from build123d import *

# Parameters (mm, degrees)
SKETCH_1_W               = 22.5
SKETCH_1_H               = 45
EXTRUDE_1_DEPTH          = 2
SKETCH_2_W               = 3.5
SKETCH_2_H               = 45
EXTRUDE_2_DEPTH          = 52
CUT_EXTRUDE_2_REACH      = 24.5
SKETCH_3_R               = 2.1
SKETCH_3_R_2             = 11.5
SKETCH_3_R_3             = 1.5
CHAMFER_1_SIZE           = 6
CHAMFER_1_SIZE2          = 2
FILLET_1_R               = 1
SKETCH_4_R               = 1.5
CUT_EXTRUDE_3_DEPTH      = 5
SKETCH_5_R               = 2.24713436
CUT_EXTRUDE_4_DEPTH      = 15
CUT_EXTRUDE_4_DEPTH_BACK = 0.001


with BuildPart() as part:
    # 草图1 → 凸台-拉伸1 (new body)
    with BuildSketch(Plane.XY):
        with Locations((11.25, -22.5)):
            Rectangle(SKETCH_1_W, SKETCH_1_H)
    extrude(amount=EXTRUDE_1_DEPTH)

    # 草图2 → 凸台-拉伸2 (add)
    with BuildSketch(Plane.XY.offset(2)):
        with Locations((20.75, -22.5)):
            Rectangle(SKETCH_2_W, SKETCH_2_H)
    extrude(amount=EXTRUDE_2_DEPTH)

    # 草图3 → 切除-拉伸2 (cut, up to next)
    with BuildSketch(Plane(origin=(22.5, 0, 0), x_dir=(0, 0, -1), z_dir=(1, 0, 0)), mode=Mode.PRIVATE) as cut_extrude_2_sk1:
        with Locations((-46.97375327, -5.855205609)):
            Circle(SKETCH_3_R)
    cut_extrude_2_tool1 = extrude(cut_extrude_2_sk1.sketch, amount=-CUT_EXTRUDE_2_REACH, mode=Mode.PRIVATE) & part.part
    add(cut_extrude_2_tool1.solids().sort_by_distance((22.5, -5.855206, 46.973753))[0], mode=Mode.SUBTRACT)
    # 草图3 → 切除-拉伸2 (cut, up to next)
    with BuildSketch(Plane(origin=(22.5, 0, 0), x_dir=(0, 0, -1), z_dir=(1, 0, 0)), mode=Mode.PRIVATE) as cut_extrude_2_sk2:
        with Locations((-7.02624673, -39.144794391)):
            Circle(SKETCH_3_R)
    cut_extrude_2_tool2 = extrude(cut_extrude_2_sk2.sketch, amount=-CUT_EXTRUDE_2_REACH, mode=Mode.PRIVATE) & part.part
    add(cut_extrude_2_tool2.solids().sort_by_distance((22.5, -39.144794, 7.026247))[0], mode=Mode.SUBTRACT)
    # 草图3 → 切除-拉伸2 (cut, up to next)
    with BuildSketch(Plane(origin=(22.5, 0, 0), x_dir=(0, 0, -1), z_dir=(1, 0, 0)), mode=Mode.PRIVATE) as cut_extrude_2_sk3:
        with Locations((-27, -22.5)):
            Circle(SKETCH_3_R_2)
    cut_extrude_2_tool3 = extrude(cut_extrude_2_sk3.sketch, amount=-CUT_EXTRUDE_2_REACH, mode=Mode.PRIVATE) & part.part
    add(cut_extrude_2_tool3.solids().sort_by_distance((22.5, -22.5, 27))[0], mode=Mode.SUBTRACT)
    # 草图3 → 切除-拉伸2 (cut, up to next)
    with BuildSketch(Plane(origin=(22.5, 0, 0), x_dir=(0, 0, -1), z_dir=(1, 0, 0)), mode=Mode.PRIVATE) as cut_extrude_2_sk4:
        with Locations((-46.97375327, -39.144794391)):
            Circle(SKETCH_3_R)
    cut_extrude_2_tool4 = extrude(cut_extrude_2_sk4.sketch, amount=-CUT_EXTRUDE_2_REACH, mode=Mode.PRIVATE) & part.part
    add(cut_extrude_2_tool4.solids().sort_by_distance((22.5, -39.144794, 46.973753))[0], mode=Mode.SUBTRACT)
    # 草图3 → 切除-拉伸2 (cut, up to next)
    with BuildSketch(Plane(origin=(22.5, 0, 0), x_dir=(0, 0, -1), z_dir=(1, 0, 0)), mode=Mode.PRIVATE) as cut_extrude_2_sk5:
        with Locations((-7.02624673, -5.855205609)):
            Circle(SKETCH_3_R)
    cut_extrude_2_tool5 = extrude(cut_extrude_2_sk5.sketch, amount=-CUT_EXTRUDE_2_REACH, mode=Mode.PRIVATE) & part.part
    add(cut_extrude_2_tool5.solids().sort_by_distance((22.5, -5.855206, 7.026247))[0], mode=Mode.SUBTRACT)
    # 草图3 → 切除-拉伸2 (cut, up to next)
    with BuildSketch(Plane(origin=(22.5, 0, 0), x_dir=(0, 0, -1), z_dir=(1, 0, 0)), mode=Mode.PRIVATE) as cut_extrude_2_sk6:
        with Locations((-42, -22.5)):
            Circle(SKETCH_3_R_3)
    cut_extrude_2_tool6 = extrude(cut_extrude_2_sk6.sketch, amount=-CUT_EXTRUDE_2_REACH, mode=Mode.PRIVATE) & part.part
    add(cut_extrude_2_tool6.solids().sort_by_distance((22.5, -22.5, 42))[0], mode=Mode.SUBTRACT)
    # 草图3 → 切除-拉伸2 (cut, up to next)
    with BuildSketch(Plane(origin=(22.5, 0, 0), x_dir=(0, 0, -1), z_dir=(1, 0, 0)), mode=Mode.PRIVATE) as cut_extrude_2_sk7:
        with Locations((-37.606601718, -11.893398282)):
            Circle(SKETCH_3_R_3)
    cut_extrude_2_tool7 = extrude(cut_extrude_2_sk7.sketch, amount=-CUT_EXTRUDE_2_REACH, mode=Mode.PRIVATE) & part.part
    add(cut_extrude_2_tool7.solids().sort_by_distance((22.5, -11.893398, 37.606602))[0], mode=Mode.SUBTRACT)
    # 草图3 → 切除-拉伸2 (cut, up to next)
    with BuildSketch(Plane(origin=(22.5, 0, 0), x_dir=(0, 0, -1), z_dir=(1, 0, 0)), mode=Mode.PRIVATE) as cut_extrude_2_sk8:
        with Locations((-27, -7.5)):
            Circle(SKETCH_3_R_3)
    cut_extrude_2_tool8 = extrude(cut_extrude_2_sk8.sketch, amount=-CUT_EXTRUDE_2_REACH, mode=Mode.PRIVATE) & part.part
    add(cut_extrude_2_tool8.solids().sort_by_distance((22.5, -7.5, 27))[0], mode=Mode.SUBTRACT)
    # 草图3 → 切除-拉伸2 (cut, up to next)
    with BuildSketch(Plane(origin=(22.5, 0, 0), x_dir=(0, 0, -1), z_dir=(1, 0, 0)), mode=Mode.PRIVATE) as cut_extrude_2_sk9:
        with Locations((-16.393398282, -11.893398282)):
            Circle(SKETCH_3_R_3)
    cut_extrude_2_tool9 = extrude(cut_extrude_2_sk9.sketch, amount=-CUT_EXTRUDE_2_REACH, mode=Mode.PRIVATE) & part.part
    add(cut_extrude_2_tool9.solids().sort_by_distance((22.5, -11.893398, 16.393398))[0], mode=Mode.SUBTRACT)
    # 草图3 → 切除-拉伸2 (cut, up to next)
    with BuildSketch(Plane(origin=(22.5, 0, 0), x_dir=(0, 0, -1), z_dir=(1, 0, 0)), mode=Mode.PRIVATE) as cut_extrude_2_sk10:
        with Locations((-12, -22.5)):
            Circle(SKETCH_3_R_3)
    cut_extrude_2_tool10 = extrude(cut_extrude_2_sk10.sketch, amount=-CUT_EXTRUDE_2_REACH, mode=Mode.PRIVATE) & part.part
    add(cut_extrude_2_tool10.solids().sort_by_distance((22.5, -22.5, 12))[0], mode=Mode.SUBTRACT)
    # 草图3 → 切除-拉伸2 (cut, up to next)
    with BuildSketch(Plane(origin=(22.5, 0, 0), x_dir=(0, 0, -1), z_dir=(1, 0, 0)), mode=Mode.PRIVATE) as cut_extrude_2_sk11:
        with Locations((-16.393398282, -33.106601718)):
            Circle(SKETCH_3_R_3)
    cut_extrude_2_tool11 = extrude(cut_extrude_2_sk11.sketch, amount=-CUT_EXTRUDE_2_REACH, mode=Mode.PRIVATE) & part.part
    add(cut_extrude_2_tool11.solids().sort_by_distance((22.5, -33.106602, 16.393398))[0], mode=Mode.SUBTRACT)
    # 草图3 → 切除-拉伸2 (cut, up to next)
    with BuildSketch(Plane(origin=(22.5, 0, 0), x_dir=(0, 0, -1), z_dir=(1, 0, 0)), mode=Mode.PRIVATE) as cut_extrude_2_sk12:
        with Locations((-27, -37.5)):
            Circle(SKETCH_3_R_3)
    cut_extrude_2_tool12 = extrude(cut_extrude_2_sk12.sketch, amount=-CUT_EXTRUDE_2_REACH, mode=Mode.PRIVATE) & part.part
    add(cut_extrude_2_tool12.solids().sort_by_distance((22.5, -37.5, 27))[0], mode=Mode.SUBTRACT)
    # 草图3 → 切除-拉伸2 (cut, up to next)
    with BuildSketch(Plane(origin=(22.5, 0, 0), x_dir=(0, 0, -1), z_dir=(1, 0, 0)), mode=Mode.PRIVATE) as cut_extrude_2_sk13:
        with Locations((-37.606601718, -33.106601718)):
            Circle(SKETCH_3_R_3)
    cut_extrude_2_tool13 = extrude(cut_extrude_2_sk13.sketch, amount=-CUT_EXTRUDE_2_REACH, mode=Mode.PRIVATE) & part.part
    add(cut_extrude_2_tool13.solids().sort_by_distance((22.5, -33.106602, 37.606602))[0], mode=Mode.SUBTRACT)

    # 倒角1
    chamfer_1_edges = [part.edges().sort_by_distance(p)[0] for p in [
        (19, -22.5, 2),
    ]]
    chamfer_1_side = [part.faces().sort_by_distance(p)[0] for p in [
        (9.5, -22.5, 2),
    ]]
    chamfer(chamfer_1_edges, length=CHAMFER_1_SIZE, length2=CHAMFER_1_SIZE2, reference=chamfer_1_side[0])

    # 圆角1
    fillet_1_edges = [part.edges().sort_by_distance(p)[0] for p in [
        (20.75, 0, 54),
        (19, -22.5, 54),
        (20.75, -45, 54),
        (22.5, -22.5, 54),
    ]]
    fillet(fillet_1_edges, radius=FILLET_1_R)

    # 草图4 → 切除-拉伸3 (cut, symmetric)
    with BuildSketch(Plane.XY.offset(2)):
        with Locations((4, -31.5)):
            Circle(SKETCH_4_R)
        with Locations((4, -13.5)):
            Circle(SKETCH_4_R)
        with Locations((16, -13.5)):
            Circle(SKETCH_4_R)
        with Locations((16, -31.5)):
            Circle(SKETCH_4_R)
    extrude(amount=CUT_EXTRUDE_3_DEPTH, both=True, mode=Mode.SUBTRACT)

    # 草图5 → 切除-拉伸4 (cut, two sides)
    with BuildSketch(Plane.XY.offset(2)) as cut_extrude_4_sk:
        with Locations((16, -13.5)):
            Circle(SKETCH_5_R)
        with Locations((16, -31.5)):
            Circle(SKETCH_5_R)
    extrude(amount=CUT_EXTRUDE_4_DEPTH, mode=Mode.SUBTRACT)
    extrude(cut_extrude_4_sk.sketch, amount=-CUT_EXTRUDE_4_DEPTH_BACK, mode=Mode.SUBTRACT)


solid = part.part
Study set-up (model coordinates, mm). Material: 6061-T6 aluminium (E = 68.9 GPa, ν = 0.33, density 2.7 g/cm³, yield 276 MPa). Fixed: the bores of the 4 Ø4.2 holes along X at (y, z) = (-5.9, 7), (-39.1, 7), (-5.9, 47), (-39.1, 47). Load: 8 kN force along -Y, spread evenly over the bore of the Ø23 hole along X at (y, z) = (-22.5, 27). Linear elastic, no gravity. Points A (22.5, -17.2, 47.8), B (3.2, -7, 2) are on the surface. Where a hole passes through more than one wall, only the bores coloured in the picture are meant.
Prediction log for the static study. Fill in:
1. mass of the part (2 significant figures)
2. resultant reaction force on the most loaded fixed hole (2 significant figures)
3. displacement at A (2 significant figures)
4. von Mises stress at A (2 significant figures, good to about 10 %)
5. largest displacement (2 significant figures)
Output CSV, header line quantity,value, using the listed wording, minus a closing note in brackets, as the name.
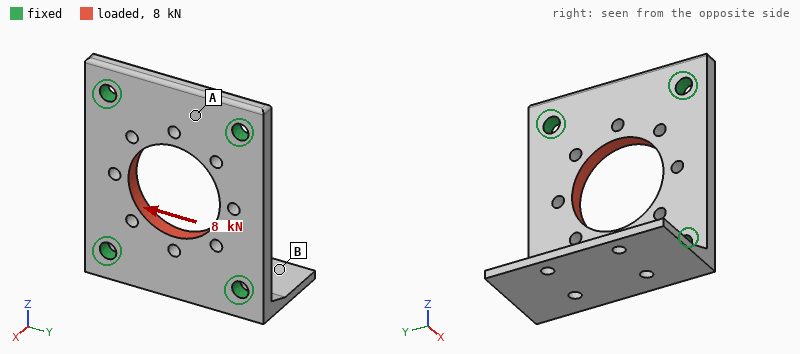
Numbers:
quantity,value
mass of the part,23 g
resultant reaction force on the most loaded fixed hole,2.2 kN
displacement at A,4.3 µm
von Mises stress at A,26 MPa
largest displacement,29 µm
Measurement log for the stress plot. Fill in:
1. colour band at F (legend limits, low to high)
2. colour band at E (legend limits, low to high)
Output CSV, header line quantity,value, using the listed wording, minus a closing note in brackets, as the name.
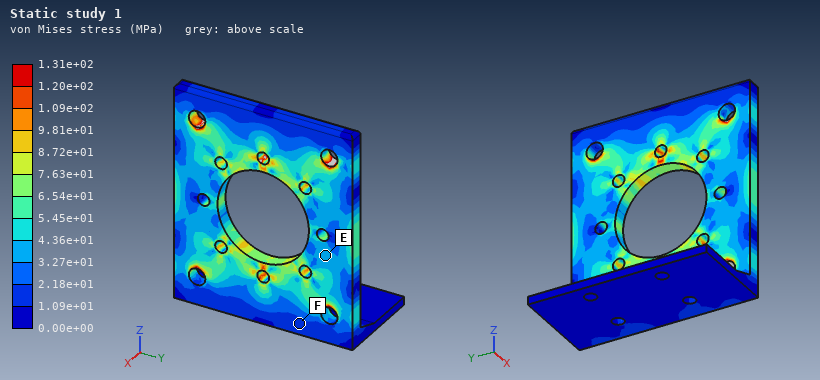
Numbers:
quantity,value
colour band at F,1.09e+01 to 2.18e+01 MPa
colour band at E,3.27e+01 to 4.36e+01 MPa
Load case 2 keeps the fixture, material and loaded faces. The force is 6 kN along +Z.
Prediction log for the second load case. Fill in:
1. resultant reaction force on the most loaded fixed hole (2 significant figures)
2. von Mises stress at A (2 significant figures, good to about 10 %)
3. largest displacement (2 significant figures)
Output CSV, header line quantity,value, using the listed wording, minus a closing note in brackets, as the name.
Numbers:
quantity,value
resultant reaction force on the most loaded fixed hole,1.6 kN
von Mises stress at A,17 MPa
largest displacement,13 µm
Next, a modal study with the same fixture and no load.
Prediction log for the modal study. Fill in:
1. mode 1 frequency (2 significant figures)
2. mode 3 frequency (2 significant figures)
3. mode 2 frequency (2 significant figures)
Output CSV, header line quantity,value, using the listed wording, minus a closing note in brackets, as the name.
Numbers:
quantity,value
mode 1 frequency,5200 Hz
mode 3 frequency,12 kHz
mode 2 frequency,7200 Hz
